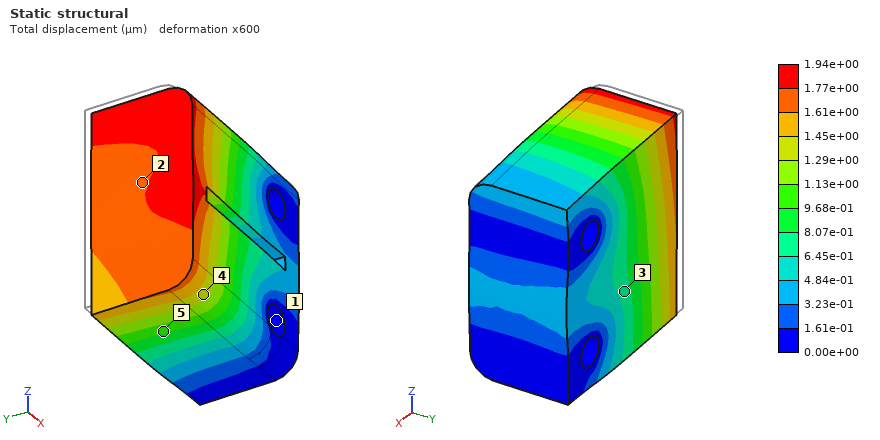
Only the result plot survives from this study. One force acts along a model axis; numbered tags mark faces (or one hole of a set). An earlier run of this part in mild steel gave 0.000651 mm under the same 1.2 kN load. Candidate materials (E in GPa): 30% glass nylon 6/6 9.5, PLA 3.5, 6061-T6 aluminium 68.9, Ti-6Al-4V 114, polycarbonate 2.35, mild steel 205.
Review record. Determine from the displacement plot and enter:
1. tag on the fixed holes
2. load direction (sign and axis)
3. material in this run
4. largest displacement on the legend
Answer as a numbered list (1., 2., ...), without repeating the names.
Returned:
1. 1
2. +X
3. 6061-T6 aluminium
4. 1.94e+00 µm
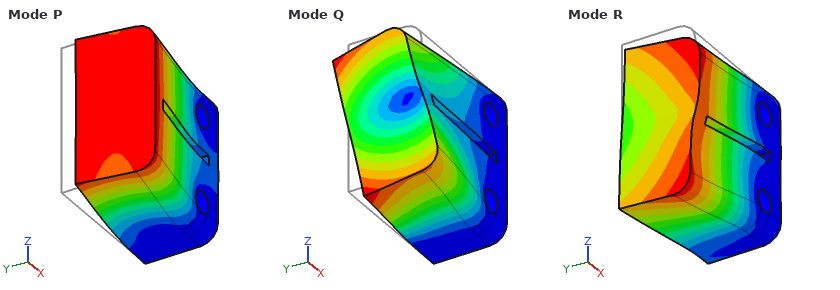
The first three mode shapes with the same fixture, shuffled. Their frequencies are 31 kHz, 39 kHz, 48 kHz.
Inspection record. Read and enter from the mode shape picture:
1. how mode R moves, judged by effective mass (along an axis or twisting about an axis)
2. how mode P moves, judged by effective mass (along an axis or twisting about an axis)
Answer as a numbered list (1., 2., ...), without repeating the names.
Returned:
1. along Z
2. along Y
